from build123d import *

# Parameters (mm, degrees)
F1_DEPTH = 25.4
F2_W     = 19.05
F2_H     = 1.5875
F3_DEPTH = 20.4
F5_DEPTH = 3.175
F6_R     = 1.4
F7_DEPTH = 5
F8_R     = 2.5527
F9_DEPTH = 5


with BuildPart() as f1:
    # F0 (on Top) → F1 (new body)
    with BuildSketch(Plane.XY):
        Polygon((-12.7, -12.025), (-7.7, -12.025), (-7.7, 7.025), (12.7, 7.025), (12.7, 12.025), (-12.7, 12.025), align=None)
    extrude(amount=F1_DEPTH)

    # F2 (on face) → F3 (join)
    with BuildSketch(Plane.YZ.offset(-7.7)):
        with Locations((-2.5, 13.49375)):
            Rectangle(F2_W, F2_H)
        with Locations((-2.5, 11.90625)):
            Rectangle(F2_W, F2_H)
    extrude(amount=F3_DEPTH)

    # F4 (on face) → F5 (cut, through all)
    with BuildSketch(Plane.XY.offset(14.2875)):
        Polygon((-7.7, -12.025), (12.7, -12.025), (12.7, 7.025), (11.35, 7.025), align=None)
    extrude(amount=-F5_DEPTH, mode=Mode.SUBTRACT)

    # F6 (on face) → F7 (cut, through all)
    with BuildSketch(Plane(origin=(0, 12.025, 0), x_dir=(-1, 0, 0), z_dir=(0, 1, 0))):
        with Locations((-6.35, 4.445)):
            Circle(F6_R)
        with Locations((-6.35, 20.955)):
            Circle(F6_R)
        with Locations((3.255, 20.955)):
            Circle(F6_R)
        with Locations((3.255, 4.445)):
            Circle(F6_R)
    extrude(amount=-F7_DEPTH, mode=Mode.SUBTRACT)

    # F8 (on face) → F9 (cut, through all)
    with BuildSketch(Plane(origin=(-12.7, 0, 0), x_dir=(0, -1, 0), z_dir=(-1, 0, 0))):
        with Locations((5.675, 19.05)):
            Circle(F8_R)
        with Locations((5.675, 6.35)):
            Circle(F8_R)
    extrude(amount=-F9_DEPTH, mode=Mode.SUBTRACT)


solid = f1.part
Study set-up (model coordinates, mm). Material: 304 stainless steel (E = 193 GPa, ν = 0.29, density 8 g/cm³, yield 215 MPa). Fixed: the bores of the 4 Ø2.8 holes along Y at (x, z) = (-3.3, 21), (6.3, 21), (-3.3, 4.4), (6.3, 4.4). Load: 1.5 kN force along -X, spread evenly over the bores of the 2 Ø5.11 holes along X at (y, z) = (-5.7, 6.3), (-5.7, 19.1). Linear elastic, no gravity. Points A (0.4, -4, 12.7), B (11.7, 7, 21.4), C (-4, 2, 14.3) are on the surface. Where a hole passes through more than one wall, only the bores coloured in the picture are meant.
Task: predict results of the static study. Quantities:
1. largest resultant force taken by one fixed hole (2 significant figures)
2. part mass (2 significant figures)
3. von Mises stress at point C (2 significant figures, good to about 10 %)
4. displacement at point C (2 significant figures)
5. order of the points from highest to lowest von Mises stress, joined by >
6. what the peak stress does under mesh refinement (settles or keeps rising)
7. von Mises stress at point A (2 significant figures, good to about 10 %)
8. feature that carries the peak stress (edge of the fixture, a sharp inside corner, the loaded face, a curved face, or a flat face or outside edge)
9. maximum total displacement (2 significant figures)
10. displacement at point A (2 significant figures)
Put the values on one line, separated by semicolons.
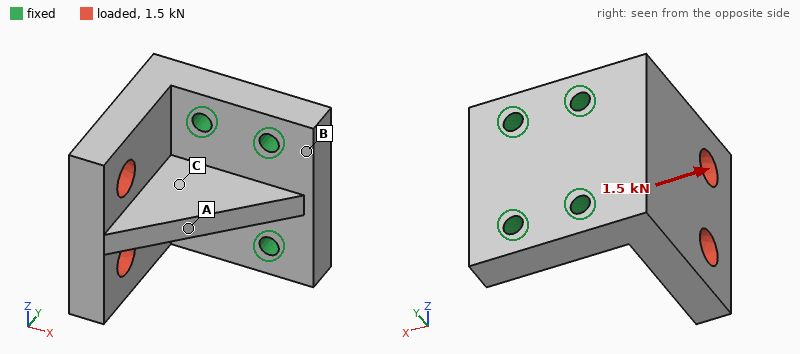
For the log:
790 N; 47 g; 46 MPa; 6.2 µm; A > C > B; keeps rising; 70 MPa; edge of the fixture; 26 µm; 11 µm
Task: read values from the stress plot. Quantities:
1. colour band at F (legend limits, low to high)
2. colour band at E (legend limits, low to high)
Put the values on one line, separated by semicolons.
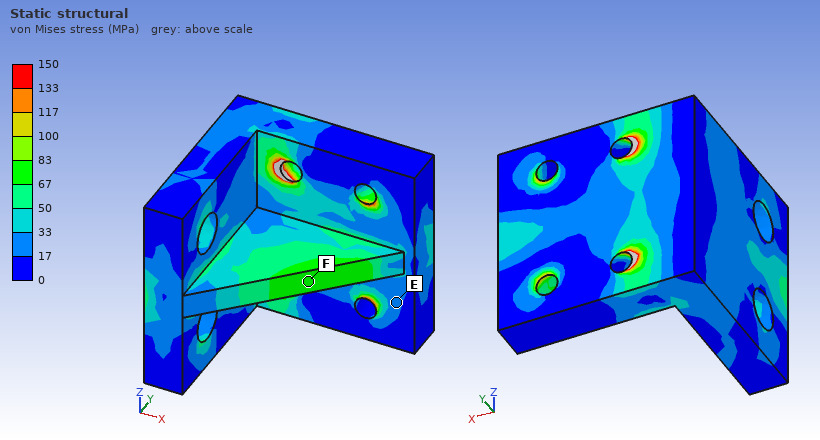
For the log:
67 to 83 MPa; 17 to 33 MPa
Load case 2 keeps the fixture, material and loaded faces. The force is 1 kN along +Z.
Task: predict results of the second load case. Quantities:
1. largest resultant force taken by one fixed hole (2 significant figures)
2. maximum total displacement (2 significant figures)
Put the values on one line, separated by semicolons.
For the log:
1.0 kN; 12 µm
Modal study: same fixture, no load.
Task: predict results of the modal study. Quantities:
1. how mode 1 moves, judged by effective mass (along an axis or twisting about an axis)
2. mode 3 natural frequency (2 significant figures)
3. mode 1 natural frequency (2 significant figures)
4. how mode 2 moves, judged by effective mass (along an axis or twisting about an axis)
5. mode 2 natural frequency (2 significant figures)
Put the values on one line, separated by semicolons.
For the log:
along X; 17 kHz; 12 kHz; along Z; 13 kHz
